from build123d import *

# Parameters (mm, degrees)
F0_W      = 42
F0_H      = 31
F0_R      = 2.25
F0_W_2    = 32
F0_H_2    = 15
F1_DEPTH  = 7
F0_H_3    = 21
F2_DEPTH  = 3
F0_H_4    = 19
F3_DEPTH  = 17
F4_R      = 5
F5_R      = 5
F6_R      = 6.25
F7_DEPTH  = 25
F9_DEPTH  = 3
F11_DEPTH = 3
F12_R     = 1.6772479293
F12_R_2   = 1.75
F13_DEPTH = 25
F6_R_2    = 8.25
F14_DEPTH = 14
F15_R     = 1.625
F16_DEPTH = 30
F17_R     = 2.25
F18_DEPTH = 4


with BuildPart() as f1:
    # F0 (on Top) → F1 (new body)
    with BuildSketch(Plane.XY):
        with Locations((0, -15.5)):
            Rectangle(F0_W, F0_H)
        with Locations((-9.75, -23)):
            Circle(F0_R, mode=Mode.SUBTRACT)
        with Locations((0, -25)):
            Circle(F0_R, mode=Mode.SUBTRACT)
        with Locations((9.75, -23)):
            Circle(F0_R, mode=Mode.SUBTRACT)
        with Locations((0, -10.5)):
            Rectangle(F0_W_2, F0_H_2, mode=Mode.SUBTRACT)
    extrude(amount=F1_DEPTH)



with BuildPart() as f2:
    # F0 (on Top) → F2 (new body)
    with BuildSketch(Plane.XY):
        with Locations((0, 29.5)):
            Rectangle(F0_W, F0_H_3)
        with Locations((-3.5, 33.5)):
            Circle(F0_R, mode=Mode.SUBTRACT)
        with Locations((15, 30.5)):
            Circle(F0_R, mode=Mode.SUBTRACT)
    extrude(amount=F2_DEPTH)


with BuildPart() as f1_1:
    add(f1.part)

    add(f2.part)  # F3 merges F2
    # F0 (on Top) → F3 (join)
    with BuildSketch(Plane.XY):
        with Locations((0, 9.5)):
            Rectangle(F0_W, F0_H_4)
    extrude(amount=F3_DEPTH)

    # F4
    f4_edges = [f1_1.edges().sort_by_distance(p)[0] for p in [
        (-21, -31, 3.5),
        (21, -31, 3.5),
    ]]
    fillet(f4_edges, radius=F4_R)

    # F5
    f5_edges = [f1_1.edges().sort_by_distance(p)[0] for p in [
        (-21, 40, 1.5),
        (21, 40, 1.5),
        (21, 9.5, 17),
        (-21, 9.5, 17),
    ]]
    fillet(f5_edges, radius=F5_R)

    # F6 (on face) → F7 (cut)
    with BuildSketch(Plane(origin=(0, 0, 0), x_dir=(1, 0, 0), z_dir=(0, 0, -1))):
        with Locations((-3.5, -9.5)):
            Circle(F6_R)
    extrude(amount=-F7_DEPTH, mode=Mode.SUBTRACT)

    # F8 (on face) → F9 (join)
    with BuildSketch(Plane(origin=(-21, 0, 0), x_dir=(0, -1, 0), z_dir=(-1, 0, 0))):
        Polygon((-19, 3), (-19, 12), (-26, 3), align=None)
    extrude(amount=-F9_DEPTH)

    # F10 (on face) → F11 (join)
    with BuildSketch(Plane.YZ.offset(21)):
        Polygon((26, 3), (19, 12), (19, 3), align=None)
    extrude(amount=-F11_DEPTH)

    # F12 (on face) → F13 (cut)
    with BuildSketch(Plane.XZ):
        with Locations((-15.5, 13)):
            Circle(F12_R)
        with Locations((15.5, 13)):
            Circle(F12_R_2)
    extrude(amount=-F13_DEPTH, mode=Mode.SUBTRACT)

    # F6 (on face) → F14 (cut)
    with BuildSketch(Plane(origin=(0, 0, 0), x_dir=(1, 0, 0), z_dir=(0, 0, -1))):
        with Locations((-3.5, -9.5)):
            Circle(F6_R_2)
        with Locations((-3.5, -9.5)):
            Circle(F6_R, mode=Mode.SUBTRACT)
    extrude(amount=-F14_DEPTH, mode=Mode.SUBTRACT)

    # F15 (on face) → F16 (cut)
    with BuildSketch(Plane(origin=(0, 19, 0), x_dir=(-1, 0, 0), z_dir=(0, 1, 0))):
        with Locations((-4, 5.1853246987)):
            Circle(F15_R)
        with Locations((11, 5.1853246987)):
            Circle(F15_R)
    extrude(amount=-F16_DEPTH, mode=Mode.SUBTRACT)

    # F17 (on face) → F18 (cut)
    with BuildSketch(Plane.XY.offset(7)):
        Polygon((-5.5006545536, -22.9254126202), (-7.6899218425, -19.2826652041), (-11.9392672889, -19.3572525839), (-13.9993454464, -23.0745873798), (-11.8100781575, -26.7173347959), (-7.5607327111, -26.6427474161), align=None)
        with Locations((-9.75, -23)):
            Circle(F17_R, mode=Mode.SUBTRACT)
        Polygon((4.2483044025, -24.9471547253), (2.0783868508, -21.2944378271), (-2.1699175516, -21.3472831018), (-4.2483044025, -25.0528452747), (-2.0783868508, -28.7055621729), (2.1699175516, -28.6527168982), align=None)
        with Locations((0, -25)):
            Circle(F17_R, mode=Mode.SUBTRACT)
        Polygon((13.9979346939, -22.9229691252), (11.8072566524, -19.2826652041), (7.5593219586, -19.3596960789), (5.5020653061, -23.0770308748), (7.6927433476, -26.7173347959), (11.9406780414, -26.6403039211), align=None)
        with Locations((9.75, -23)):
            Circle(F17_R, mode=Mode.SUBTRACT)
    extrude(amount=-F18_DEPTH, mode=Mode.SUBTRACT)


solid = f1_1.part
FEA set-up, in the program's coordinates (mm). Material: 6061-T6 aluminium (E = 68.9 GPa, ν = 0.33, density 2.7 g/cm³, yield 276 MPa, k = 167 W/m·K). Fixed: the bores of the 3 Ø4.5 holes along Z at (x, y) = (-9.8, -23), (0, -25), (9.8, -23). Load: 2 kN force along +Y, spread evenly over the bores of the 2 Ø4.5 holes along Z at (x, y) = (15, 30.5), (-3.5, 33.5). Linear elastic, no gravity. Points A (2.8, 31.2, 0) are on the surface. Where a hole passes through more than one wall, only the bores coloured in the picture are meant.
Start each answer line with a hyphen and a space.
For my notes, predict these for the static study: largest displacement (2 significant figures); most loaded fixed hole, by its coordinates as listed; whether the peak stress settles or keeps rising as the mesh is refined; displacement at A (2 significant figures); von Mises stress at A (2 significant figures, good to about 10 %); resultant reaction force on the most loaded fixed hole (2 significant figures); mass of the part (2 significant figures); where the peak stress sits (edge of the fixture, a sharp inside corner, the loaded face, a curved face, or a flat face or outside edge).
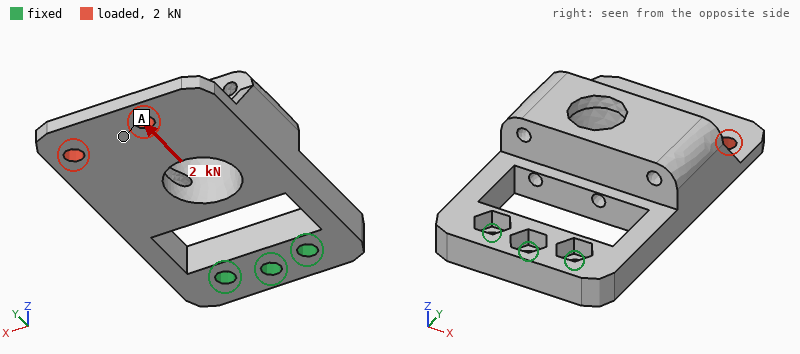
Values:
- 0.29 mm
- (9.8, -23)
- keeps rising
- 0.24 mm
- 14 MPa
- 1.6 kN
- 46 g
- edge of the fixture
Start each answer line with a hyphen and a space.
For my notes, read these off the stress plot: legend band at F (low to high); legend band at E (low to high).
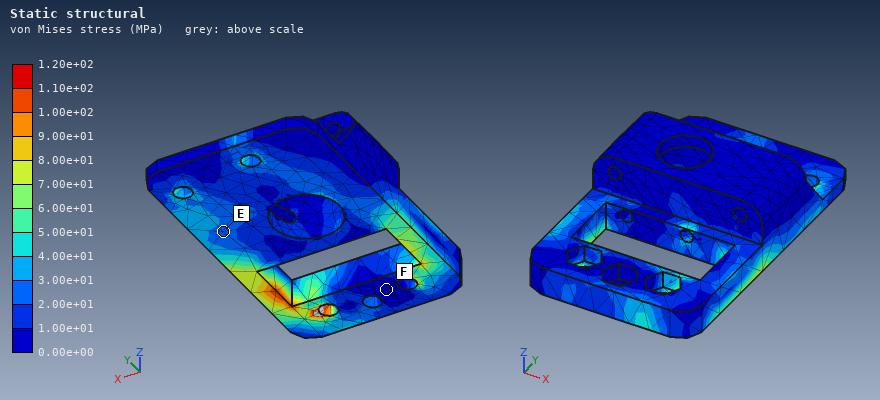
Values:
- 0.00e+00 to 1.00e+01 MPa
- 2.00e+01 to 3.00e+01 MPa
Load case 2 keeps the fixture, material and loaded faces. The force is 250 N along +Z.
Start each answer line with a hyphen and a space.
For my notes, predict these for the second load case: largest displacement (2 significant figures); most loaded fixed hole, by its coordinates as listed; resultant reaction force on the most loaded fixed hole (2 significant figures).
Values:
- 0.97 mm
- (9.8, -23)
- 350 N
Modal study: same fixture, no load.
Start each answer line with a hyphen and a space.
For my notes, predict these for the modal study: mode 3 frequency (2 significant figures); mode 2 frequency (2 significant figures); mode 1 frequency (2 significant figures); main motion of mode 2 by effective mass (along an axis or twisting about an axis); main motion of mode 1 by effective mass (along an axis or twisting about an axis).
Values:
- 3000 Hz
- 2200 Hz
- 750 Hz
- along X
- along Z
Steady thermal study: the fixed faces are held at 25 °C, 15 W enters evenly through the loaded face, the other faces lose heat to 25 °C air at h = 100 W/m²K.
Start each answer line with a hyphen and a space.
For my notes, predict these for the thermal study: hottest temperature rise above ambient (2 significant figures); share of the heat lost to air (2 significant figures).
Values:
- 26 K
- 69 %
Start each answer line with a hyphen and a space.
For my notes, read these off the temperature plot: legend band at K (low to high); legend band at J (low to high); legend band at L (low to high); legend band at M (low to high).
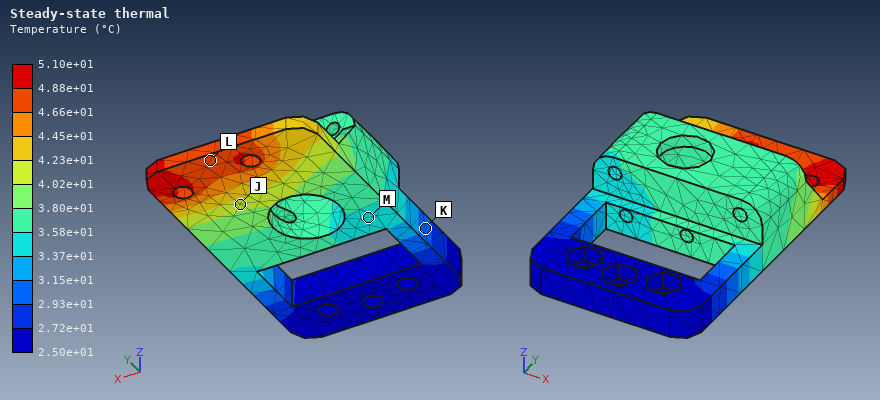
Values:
- 2.93e+01 to 3.15e+01 °C
- 4.02e+01 to 4.23e+01 °C
- 4.66e+01 to 4.88e+01 °C
- 3.37e+01 to 3.58e+01 °C
